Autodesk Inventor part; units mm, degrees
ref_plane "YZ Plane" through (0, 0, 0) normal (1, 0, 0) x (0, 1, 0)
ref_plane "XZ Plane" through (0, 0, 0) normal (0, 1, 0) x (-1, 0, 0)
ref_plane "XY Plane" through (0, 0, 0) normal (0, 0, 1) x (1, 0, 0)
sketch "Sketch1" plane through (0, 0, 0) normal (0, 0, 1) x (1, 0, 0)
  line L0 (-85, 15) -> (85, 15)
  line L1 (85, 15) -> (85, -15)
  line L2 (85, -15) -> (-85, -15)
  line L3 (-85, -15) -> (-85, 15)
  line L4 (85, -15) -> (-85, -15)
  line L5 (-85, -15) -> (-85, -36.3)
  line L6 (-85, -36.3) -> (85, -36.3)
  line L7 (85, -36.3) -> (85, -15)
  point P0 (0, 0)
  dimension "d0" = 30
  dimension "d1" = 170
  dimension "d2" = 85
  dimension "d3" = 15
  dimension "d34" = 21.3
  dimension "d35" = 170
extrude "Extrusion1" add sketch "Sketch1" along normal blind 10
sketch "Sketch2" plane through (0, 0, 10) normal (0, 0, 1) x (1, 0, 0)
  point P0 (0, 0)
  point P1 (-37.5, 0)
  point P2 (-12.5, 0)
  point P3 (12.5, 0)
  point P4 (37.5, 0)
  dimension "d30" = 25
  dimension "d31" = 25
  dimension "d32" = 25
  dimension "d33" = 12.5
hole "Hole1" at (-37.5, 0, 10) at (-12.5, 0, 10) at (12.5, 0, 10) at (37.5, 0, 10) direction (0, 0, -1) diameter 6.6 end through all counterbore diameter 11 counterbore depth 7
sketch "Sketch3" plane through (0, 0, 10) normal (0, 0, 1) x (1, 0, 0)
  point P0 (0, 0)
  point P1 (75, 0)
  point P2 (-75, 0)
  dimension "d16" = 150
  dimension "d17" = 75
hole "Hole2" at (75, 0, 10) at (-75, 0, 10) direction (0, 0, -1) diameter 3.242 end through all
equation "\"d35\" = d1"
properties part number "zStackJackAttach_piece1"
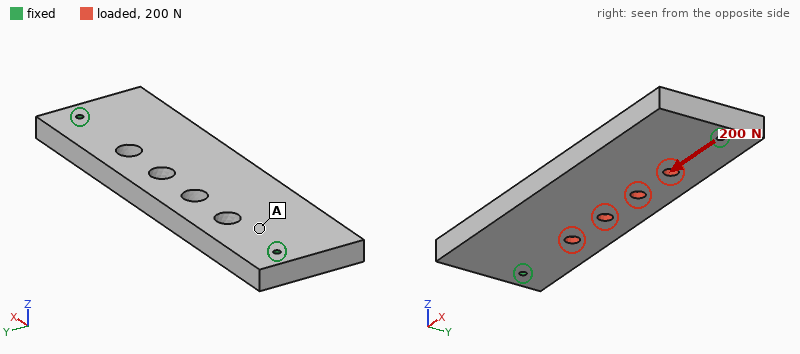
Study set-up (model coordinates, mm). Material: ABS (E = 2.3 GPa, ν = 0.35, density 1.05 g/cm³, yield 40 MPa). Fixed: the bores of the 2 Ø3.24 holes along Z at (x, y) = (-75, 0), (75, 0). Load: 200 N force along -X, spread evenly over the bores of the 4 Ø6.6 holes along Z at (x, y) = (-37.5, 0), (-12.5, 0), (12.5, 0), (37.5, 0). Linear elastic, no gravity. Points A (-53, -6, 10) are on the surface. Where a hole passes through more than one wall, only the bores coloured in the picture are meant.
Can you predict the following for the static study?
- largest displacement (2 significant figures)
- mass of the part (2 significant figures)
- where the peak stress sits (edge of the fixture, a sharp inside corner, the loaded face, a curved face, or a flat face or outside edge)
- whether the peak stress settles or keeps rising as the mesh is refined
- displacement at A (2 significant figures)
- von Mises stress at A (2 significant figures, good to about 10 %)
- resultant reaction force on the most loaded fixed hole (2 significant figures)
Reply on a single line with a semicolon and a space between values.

13 µm; 88 g; edge of the fixture; keeps rising; 6.3 µm; 0.23 MPa; 100 N
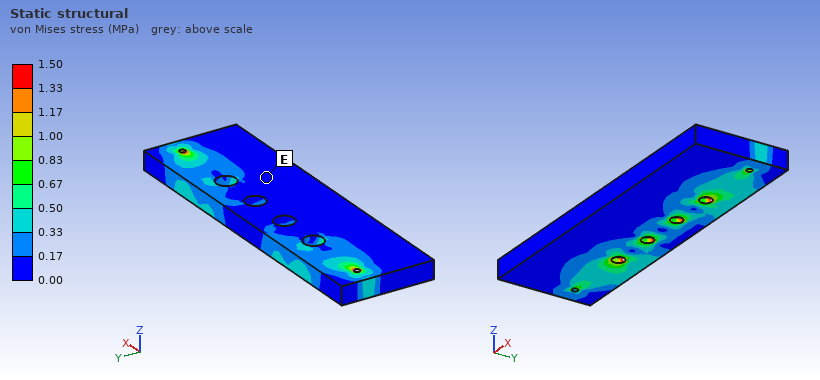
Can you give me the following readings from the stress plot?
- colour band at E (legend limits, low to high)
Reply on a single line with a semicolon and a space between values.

0.00 to 0.17 MPa
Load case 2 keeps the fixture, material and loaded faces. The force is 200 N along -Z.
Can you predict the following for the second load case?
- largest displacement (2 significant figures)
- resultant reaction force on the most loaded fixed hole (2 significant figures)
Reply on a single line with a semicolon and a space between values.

0.50 mm; 100 N
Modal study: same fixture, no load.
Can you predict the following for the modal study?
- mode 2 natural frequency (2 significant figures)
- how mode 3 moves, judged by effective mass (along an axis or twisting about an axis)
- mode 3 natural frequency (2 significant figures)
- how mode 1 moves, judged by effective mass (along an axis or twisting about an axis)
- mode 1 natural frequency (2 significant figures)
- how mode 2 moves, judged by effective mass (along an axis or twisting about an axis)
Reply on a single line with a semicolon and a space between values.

860 Hz; twisting about Y; 1200 Hz; along Z; 480 Hz; twisting about X
